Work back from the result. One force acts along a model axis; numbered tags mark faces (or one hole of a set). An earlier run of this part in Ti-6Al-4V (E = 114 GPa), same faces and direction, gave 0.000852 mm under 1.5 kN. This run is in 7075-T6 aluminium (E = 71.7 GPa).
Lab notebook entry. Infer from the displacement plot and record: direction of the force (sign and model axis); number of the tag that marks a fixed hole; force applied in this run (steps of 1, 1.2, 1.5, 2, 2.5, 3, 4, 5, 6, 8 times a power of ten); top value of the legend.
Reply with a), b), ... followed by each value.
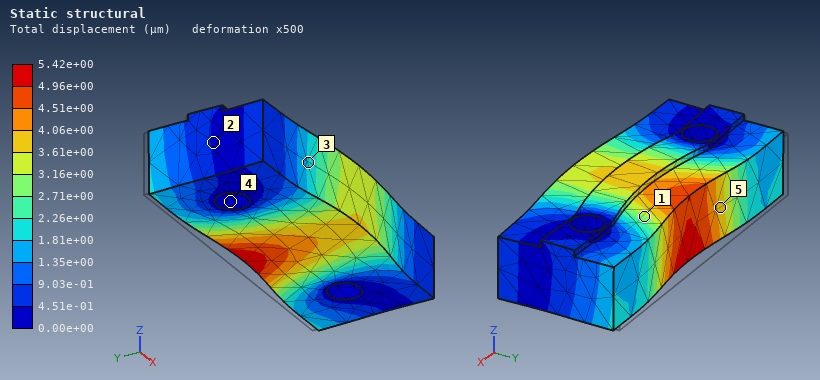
a) -Y
b) 4
c) 6 kN
d) 5.42e+00 µm
